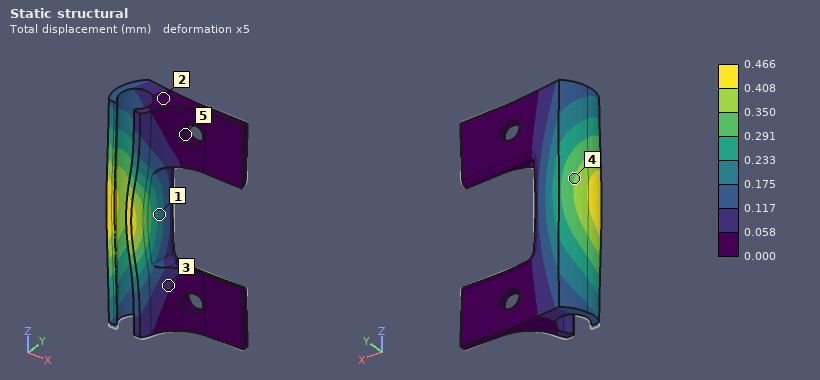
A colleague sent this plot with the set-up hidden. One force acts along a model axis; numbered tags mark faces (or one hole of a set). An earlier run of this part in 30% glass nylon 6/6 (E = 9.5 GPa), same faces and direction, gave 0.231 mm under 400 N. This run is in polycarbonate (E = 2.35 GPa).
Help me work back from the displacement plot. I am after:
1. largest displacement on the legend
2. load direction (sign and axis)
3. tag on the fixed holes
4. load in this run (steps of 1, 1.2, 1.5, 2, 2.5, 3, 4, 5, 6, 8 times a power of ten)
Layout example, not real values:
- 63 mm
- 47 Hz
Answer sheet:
- 0.466 mm
- -X
- 5
- 200 N
